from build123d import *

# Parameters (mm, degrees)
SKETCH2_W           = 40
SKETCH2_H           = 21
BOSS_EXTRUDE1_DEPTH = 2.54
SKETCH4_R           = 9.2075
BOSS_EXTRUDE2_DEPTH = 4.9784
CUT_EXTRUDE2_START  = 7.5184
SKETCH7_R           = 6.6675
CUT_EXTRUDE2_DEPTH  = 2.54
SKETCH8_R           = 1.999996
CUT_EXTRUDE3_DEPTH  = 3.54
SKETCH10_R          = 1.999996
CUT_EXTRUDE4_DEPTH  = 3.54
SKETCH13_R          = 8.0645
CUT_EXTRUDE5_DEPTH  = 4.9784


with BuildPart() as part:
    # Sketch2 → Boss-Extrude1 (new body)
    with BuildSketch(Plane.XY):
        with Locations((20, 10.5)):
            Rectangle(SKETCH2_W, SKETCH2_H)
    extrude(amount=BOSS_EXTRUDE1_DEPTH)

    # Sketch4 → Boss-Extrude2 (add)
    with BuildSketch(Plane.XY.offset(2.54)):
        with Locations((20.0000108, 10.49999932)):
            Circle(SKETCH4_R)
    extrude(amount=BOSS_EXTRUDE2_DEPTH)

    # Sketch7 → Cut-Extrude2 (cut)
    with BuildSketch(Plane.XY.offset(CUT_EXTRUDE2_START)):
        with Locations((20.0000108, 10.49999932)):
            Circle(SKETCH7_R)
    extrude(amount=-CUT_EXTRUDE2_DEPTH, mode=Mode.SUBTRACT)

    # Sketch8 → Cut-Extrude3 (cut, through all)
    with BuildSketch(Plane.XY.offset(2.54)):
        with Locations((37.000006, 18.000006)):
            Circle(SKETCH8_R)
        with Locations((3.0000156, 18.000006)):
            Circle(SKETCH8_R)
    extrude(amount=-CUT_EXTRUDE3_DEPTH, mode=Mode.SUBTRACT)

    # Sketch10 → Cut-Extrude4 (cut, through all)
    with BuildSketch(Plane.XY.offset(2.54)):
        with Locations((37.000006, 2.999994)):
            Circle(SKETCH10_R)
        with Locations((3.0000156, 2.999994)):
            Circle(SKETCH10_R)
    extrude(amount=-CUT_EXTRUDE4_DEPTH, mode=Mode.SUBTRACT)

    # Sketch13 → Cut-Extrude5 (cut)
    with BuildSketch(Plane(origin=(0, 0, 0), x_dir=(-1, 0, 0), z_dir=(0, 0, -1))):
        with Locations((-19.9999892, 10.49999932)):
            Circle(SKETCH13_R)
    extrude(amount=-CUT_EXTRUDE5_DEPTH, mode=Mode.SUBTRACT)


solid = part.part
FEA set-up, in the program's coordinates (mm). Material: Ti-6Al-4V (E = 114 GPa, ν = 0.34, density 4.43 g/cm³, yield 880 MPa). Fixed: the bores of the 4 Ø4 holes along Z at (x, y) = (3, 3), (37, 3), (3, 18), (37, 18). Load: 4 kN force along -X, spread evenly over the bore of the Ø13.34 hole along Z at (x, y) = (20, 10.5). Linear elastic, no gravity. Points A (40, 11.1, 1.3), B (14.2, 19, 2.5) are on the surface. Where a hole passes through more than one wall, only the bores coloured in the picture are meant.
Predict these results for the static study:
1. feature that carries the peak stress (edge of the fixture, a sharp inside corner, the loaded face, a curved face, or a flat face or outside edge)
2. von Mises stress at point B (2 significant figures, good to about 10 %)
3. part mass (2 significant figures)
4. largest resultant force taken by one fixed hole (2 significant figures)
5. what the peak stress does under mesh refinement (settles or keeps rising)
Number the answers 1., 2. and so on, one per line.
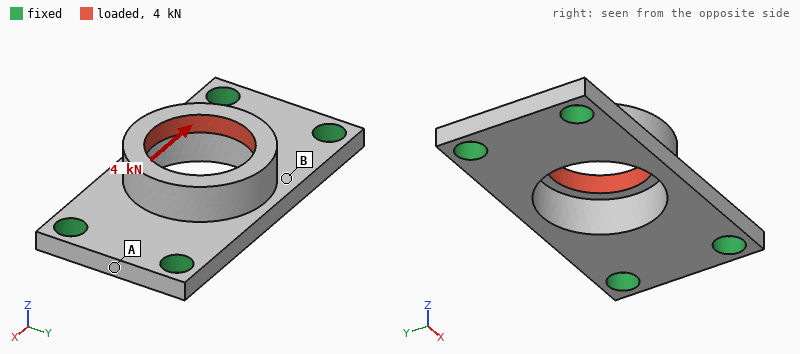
1. edge of the fixture
2. 150 MPa
3. 8.7 g
4. 1.1 kN
5. keeps rising
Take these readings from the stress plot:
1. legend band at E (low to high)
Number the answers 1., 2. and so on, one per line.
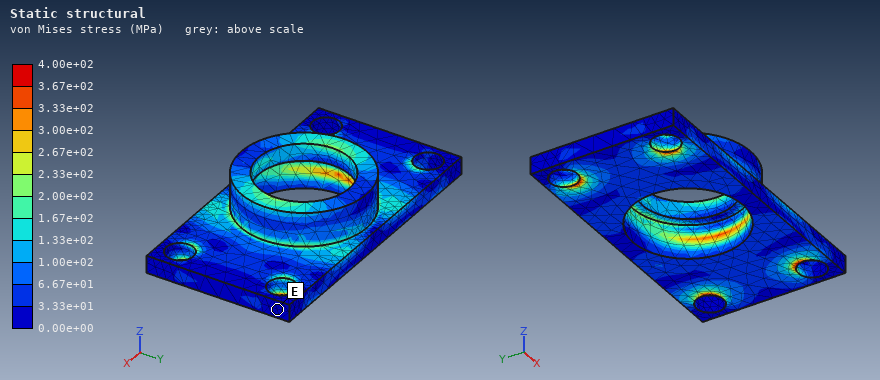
1. 0.00e+00 to 3.33e+01 MPa
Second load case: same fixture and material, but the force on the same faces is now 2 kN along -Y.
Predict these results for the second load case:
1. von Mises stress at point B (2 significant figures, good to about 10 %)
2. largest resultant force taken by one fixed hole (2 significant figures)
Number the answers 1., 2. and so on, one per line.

1. 94 MPa
2. 730 N
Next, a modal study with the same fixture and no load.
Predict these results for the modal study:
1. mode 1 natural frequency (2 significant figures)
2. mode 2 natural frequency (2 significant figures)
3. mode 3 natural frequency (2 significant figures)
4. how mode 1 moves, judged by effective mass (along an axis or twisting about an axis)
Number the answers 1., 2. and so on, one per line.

1. 15 kHz
2. 16 kHz
3. 27 kHz
4. along Z
